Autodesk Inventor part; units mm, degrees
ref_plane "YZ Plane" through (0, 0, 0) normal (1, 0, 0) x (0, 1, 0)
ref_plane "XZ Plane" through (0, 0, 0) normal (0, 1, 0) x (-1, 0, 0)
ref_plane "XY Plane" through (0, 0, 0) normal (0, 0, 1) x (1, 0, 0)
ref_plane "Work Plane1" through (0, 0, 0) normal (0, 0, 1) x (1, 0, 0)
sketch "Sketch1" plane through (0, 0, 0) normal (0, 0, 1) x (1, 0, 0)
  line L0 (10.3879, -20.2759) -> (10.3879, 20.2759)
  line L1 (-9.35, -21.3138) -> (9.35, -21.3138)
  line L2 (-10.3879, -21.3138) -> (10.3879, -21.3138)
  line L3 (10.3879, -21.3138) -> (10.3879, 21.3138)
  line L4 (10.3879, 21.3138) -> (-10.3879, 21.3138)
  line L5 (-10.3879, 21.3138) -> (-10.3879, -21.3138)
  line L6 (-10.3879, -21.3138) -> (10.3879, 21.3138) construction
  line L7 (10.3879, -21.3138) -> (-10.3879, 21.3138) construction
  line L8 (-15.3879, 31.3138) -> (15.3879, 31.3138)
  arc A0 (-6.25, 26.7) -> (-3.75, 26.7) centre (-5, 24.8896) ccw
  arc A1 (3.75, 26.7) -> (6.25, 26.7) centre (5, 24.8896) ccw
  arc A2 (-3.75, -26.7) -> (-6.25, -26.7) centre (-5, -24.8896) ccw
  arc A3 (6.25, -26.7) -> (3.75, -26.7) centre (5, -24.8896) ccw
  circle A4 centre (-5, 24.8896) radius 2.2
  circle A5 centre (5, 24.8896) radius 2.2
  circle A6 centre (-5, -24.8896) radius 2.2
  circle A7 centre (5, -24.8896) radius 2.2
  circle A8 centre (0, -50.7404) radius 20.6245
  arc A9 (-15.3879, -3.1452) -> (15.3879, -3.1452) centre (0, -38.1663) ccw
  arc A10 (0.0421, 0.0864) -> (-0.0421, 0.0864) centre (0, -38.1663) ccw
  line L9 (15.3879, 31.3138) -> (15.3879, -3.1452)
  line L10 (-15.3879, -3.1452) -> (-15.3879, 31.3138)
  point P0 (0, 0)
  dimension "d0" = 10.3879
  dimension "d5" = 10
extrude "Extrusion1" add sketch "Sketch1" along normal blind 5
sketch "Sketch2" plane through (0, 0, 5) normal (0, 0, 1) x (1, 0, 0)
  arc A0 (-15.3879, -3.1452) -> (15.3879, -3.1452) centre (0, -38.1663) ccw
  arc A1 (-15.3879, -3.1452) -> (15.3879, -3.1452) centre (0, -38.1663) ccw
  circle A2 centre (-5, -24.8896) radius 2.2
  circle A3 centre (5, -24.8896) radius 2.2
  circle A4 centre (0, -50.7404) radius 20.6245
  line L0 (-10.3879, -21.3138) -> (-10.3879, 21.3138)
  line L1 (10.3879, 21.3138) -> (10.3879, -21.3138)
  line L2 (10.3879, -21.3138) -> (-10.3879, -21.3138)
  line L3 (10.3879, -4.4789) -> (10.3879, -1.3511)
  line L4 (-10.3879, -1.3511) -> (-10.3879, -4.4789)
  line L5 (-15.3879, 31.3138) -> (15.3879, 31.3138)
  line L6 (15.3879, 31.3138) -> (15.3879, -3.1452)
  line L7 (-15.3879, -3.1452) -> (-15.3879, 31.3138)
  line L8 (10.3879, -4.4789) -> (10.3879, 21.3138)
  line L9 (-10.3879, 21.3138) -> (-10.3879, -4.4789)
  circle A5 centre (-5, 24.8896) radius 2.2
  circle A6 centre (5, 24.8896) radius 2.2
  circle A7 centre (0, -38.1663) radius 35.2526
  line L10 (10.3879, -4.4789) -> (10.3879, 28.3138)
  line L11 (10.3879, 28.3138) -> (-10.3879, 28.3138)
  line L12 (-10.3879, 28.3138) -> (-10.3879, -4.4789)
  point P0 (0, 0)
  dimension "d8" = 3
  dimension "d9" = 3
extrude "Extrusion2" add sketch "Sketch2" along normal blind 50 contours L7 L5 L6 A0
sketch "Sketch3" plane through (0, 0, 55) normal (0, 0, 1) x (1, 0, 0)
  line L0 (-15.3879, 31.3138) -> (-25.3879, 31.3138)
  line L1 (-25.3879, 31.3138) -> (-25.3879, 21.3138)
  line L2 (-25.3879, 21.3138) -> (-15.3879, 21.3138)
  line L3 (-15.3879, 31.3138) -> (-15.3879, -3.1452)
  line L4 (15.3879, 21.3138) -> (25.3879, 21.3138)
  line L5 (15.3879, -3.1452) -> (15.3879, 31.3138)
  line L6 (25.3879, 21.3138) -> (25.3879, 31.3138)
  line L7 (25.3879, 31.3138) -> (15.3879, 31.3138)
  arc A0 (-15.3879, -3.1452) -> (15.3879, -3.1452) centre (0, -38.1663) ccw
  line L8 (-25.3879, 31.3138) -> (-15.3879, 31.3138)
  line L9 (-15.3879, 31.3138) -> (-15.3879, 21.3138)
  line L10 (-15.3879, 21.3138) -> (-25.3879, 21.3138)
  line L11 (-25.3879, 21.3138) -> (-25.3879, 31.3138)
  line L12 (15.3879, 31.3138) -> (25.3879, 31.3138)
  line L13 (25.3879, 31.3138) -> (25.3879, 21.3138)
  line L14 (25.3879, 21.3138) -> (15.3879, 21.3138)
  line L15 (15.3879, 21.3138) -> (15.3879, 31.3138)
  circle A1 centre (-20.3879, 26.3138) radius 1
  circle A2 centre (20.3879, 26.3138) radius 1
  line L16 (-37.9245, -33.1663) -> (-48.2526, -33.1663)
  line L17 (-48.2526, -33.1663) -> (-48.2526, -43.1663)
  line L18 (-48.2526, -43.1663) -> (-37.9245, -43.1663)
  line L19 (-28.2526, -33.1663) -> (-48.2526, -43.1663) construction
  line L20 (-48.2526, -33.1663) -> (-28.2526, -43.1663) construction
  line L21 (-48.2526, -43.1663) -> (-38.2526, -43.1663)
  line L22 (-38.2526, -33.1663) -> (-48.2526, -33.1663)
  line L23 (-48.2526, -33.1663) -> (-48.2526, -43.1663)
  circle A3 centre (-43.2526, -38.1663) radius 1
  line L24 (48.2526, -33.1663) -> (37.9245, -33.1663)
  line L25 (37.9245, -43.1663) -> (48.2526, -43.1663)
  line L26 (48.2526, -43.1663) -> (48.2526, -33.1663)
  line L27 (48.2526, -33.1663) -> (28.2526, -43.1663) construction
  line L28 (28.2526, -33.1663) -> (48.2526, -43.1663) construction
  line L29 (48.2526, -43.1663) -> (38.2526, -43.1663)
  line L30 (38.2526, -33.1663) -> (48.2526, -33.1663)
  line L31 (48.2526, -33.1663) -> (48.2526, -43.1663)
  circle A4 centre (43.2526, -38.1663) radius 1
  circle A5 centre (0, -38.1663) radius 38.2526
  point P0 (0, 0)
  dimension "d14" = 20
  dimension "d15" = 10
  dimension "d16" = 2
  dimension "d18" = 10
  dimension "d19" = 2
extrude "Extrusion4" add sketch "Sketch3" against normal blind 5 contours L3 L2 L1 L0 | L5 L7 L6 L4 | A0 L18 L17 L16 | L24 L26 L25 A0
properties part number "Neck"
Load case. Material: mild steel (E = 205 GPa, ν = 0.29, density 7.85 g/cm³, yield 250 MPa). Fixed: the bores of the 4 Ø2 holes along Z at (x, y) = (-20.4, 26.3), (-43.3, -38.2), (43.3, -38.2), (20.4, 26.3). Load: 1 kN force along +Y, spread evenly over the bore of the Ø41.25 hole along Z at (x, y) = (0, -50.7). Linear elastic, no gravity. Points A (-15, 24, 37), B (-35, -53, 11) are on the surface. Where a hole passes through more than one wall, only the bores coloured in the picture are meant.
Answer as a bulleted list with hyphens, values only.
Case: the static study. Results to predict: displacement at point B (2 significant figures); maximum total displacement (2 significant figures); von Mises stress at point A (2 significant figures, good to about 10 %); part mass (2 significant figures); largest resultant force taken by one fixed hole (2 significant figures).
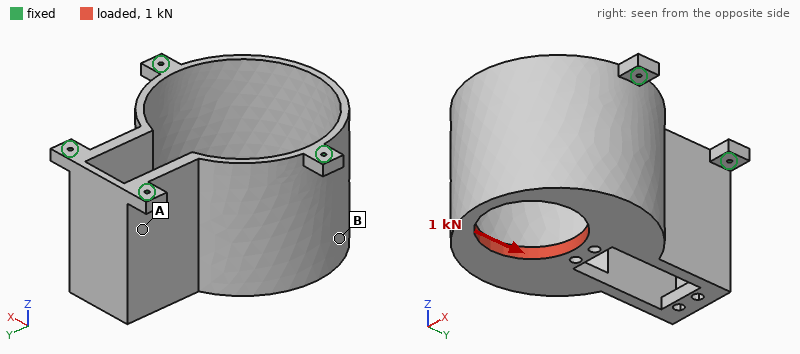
- 9.1 µm
- 15 µm
- 5.7 MPa
- 550 g
- 530 N
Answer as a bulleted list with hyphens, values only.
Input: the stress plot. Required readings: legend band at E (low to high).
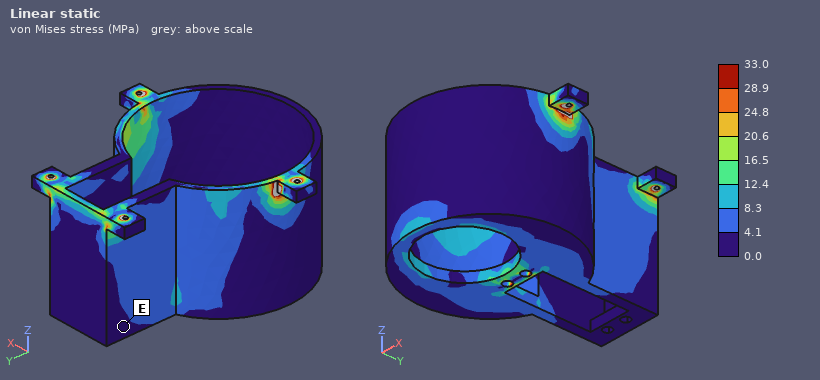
- 0.0 to 4.1 MPa
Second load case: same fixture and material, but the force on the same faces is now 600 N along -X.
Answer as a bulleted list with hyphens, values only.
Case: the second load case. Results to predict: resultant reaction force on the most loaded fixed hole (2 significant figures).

- 450 N
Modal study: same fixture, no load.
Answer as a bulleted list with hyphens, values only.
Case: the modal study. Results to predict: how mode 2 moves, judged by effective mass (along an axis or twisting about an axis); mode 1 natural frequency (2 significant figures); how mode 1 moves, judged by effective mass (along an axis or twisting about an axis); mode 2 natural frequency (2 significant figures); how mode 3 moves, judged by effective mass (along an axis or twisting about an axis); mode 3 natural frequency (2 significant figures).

- along Y
- 1800 Hz
- along X
- 2700 Hz
- along X
- 3000 Hz
